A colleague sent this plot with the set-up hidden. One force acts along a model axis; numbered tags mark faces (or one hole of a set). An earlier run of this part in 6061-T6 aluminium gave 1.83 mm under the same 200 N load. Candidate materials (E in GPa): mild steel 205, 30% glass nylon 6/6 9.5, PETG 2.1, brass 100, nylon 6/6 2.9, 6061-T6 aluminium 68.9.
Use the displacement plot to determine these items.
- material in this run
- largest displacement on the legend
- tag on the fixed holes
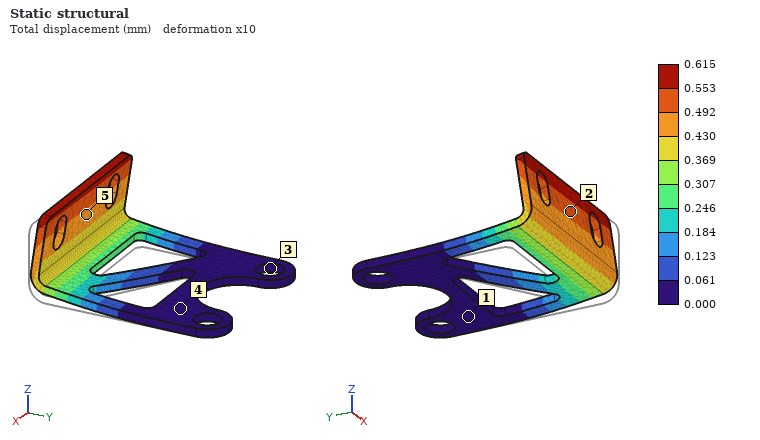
mild steel
0.615 mm
3
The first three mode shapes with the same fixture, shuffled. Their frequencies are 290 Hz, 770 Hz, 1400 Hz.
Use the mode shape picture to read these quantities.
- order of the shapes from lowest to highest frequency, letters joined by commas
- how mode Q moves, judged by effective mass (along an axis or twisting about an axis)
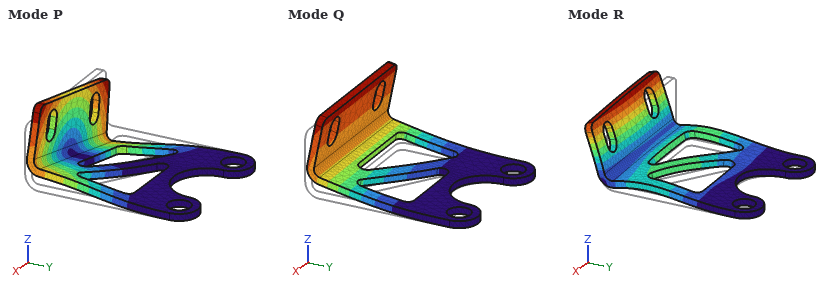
Q, P, R
along Z
